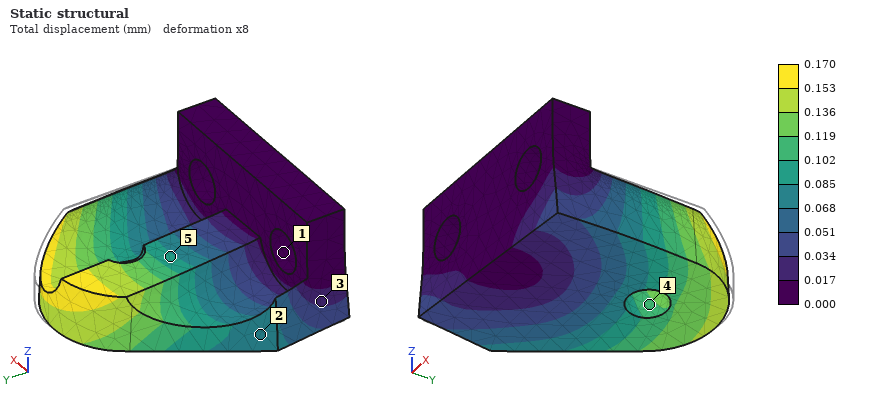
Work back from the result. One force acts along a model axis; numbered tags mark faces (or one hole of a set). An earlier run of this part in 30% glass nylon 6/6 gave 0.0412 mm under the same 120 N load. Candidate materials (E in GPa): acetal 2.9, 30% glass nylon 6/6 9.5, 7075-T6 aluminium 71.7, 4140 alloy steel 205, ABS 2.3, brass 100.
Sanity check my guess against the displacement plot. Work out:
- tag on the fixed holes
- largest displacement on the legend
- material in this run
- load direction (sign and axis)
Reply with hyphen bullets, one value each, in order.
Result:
- 1
- 0.170 mm
- ABS
- -X
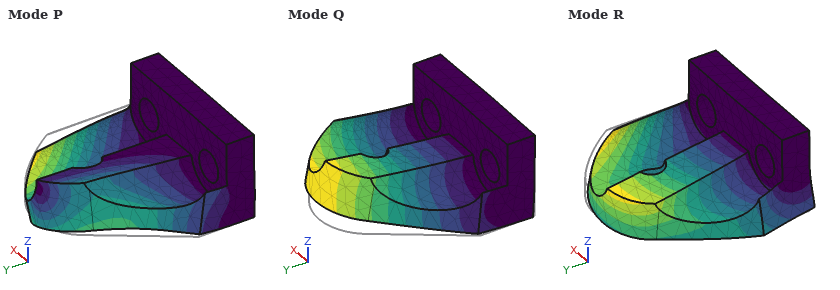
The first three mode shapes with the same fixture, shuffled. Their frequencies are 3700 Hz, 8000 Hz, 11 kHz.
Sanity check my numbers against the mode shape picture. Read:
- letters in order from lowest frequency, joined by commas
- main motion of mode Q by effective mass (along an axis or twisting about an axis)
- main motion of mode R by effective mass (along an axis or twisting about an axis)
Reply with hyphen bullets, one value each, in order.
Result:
- Q, R, P
- along Z
- along X
